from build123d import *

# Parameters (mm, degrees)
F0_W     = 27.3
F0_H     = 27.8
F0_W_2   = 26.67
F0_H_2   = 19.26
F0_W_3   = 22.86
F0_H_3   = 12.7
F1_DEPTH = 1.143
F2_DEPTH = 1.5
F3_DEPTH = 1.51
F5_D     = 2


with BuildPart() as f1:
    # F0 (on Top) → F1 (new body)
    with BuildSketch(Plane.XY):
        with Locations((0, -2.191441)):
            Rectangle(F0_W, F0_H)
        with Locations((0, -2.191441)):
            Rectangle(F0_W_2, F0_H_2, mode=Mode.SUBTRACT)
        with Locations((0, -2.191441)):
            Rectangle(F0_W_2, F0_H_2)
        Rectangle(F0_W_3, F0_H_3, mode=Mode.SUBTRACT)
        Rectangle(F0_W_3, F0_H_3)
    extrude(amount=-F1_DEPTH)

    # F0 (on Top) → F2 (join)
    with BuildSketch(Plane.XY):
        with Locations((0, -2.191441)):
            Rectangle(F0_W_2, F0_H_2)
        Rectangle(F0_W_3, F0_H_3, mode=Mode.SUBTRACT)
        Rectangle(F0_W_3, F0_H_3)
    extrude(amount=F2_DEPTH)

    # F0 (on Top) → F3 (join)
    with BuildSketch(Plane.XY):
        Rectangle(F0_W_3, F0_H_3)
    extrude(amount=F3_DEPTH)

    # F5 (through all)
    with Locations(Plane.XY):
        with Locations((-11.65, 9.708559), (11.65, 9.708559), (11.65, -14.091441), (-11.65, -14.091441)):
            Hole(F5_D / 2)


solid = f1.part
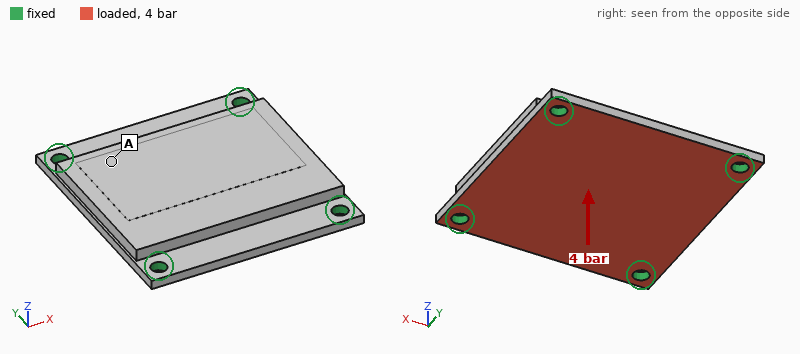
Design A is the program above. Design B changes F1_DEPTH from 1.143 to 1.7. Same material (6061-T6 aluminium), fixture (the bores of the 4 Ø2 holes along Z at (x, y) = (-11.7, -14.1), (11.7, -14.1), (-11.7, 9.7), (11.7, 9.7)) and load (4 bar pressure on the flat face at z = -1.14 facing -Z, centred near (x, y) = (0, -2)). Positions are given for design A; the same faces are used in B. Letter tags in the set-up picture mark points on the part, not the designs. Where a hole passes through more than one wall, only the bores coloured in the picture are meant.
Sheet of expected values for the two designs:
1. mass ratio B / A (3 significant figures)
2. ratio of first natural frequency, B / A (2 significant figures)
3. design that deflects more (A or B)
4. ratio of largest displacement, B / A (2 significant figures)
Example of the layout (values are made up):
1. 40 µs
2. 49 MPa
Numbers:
1. 1.26
2. 1.2
3. A
4. 0.53
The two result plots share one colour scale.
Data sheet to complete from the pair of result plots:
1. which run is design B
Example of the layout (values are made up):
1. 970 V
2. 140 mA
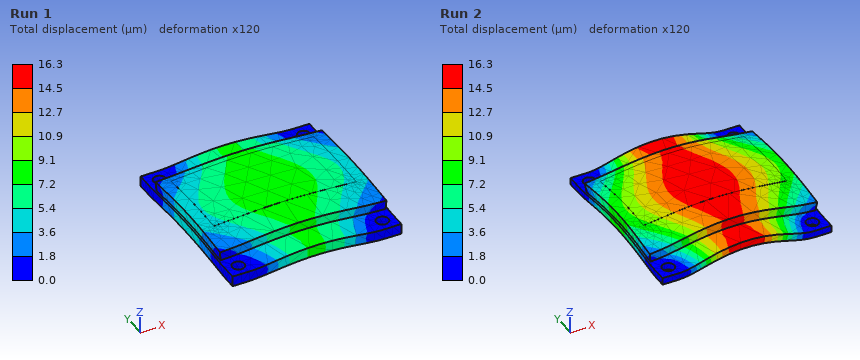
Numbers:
1. Run 1
